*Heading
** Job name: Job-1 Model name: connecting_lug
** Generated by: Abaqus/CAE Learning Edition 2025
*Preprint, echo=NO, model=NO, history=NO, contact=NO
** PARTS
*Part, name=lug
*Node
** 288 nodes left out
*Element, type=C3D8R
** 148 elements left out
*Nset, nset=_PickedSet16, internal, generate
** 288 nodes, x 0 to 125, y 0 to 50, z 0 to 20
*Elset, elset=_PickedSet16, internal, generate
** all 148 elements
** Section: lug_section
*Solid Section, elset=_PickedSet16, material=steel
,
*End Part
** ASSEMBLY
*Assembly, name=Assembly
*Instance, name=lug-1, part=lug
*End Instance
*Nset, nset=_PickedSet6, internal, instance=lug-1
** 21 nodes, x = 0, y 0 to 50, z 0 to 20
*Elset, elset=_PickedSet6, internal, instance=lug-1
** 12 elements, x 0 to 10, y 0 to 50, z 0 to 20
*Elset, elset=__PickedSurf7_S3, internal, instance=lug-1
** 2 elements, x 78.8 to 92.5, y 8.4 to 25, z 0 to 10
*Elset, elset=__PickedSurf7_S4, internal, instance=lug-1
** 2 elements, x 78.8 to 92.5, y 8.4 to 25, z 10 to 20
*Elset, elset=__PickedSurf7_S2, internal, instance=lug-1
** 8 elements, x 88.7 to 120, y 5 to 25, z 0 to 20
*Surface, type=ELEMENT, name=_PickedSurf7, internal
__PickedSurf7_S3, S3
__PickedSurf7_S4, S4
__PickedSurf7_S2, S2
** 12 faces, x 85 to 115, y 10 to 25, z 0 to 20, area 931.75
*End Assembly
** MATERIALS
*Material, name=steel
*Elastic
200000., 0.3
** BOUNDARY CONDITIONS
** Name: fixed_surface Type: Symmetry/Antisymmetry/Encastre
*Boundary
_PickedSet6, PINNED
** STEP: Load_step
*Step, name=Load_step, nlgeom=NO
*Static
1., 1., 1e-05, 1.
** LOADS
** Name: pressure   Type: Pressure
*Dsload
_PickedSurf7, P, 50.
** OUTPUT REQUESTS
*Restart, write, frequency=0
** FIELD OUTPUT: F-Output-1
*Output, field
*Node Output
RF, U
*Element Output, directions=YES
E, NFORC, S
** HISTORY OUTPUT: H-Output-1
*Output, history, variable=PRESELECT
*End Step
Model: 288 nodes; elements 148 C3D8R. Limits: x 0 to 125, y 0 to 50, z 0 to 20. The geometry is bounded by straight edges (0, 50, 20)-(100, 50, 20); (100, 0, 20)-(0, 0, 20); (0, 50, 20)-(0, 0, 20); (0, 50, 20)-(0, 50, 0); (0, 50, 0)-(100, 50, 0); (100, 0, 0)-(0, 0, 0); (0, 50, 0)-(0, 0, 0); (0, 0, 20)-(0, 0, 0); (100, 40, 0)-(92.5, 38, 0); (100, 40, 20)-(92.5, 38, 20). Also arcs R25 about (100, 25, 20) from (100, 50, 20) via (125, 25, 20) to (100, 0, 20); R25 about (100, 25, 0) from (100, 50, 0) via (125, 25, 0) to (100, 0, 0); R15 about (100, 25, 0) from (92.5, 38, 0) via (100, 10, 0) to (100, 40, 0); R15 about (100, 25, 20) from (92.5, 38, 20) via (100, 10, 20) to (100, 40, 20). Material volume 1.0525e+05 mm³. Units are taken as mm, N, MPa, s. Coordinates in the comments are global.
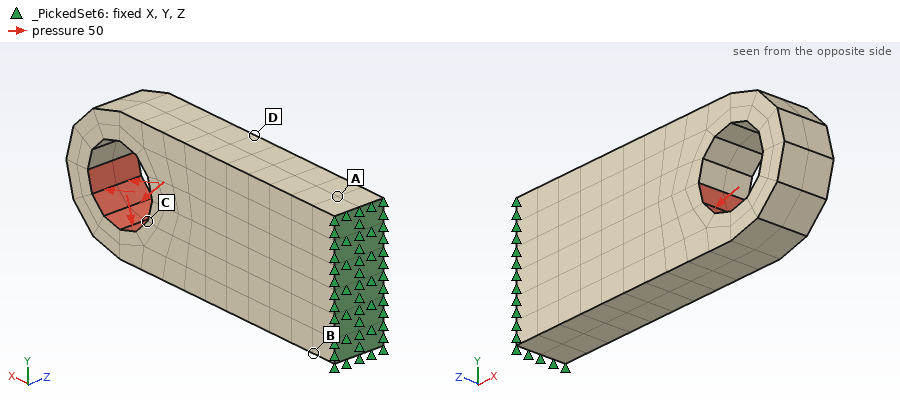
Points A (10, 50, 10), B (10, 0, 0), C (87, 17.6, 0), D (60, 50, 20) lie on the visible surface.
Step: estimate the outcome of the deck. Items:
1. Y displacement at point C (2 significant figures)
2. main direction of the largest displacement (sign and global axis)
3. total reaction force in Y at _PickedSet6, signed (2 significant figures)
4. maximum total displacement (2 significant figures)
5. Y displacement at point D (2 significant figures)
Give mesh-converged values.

-0.23 mm
-Y
30000 N
0.42 mm
-0.13 mm
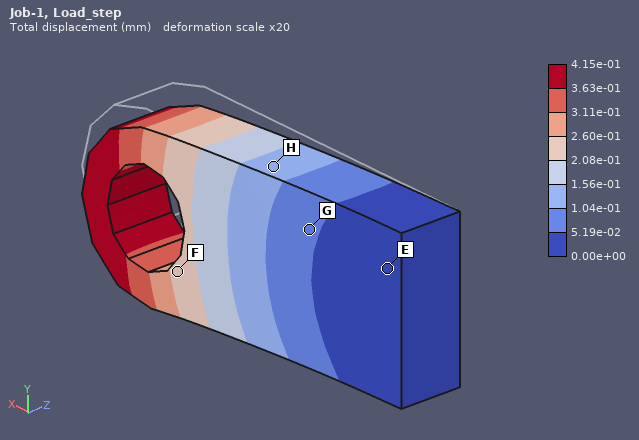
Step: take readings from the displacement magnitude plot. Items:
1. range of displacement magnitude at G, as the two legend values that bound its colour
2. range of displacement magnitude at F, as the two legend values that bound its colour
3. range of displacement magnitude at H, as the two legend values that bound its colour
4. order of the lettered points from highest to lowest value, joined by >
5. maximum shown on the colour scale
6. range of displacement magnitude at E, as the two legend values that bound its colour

5.19e-02 to 1.04e-01 mm
2.08e-01 to 2.60e-01 mm
1.04e-01 to 1.56e-01 mm
F > H > G > E
4.15e-01 mm
0.00e+00 to 5.19e-02 mm
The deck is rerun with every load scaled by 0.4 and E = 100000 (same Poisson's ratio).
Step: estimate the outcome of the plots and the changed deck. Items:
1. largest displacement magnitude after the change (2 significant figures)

0.33 mm
